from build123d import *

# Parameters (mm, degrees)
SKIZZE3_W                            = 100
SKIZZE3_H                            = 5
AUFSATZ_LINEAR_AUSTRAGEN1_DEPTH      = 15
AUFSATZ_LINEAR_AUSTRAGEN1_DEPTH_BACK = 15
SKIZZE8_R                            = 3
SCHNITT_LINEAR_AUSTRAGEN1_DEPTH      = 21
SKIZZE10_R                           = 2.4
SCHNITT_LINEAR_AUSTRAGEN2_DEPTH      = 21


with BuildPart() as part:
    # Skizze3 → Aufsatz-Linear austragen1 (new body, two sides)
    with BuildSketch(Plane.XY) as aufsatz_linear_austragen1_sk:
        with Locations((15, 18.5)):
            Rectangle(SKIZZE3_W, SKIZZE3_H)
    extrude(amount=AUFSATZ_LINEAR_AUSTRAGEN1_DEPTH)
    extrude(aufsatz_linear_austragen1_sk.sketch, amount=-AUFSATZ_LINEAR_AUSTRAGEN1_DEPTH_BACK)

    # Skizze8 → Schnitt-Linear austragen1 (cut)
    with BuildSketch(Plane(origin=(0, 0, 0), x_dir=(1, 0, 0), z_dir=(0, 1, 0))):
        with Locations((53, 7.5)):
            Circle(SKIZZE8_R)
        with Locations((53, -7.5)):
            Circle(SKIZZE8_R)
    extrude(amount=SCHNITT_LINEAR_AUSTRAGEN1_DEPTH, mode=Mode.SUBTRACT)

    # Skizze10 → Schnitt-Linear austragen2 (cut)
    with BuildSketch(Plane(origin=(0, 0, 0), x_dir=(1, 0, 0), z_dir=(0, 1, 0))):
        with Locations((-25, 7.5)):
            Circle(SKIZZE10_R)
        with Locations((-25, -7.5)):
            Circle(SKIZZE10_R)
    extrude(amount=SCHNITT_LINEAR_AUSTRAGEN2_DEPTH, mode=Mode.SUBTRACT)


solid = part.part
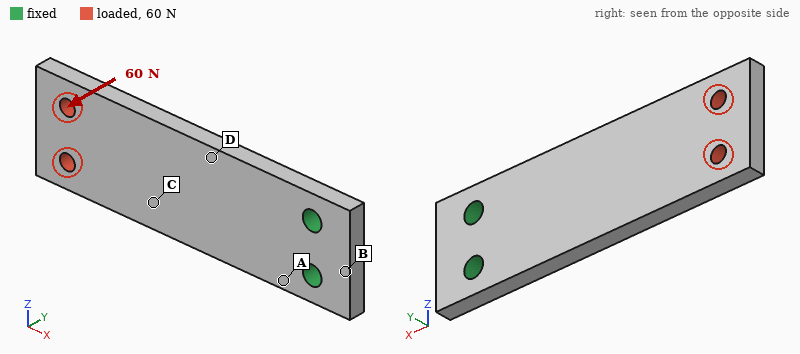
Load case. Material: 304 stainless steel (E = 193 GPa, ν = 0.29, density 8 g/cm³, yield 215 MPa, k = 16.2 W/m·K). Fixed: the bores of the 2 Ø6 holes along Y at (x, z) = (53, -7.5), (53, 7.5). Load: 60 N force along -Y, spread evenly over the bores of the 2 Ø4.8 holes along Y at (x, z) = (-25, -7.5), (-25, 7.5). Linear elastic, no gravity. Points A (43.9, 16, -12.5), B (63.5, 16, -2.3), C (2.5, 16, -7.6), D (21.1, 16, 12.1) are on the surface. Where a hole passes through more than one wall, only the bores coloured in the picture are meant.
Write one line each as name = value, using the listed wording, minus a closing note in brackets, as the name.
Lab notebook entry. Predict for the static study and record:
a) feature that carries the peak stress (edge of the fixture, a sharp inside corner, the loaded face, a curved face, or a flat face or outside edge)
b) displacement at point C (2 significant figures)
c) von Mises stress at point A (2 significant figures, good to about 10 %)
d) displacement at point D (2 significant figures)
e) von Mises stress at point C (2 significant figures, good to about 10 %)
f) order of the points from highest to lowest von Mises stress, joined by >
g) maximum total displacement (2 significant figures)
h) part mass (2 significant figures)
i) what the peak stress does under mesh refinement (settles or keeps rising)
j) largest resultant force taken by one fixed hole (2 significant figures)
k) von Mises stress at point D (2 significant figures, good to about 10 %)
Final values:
feature that carries the peak stress = edge of the fixture
displacement at point C = 0.070 mm
von Mises stress at point A = 32 MPa
displacement at point D = 0.030 mm
von Mises stress at point C = 13 MPa
order of the points from highest to lowest von Mises stress, joined by > = A > D > C > B
maximum total displacement = 0.17 mm
part mass = 120 g
what the peak stress does under mesh refinement = keeps rising
largest resultant force taken by one fixed hole = 30 N
von Mises stress at point D = 22 MPa
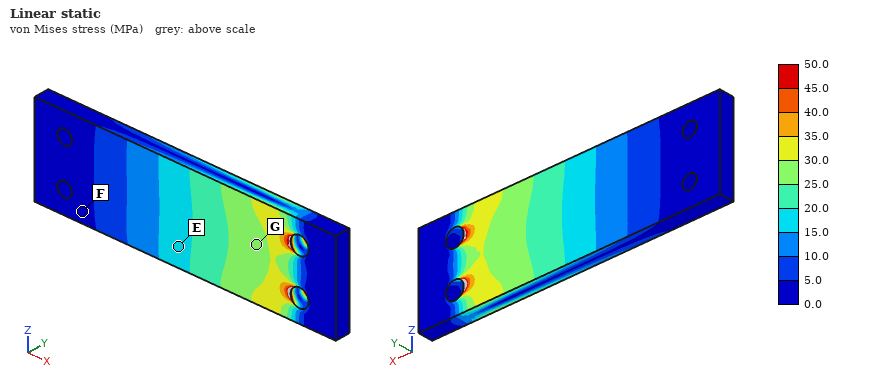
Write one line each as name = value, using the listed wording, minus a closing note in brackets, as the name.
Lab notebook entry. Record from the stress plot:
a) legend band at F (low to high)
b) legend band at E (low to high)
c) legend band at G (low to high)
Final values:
legend band at F = 0.0 to 5.0 MPa
legend band at E = 15.0 to 20.0 MPa
legend band at G = 25.0 to 30.0 MPa
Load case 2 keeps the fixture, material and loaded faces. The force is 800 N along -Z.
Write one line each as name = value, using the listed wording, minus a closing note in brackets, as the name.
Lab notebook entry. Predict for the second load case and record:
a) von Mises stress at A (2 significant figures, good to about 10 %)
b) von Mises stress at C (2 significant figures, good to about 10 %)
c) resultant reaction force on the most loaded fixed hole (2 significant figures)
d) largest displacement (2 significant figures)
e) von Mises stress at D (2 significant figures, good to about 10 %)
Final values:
von Mises stress at A = 58 MPa
von Mises stress at C = 18 MPa
resultant reaction force on the most loaded fixed hole = 3.3 kN
largest displacement = 80 µm
von Mises stress at D = 40 MPa
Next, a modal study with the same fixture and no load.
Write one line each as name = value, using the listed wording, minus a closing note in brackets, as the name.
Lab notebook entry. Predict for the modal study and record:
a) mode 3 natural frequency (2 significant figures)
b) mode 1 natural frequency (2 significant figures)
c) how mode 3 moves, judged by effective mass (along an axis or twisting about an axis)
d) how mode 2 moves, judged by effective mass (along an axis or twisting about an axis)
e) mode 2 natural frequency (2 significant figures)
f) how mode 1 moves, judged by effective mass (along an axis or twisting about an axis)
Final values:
mode 3 natural frequency = 3000 Hz
mode 1 natural frequency = 550 Hz
how mode 3 moves, judged by effective mass = twisting about X
how mode 2 moves, judged by effective mass = along Z
mode 2 natural frequency = 2800 Hz
how mode 1 moves, judged by effective mass = along Y
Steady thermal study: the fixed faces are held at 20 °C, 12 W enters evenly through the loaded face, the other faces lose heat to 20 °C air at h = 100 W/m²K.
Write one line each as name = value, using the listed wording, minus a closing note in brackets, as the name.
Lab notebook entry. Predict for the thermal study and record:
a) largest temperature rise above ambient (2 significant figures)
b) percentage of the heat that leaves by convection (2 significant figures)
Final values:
largest temperature rise above ambient = 65 K
percentage of the heat that leaves by convection = 98 %
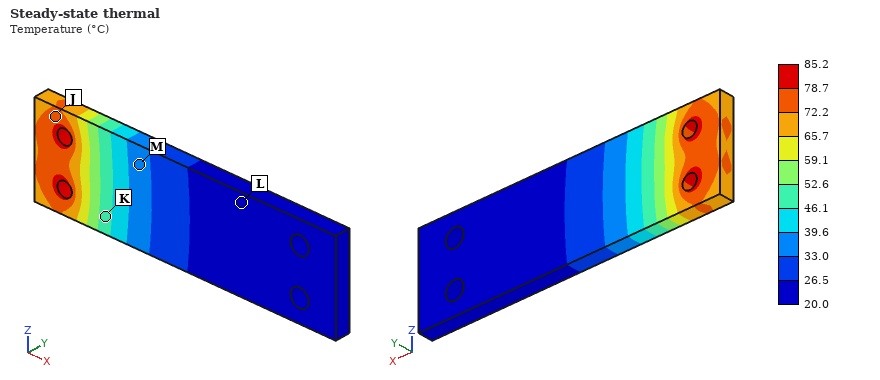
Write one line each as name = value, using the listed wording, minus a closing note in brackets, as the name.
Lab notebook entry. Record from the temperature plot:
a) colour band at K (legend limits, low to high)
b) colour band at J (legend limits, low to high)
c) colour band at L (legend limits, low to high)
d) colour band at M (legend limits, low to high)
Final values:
colour band at K = 46.1 to 52.6 °C
colour band at J = 72.2 to 78.7 °C
colour band at L = 20.0 to 26.5 °C
colour band at M = 33.0 to 39.6 °C
